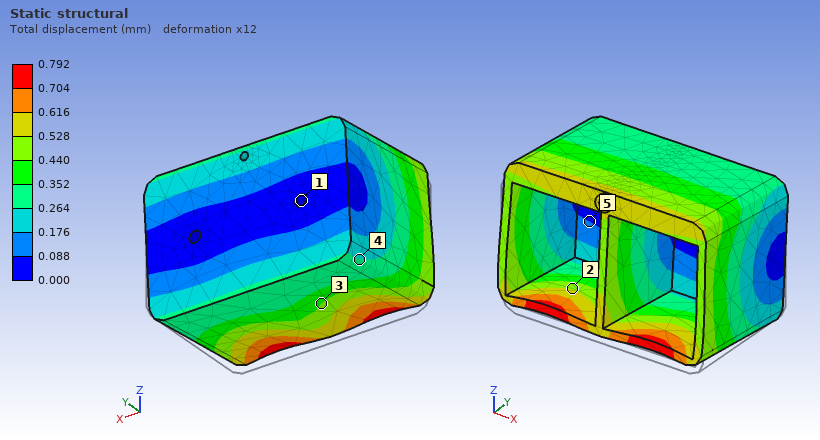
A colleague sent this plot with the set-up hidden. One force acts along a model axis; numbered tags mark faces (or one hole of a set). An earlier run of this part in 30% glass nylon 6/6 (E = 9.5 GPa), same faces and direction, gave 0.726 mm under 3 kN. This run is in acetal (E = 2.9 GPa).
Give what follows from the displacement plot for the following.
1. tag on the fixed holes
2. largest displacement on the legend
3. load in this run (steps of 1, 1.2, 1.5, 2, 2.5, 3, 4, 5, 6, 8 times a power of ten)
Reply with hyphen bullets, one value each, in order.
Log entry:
- 1
- 0.792 mm
- 1 kN
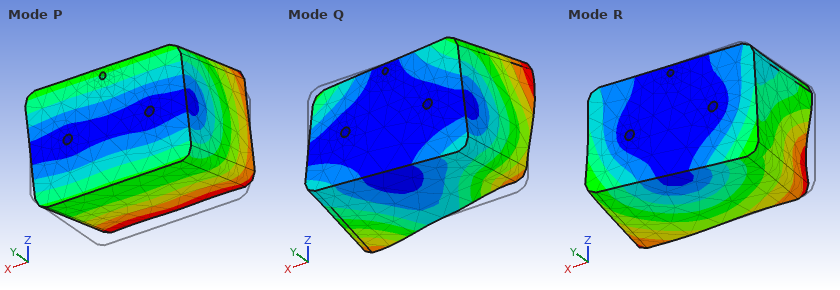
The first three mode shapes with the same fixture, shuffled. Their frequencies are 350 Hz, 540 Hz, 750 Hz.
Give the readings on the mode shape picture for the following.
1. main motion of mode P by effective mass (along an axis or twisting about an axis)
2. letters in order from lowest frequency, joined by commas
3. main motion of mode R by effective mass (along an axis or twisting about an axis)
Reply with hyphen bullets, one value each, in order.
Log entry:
- along Z
- P, Q, R
- along X
